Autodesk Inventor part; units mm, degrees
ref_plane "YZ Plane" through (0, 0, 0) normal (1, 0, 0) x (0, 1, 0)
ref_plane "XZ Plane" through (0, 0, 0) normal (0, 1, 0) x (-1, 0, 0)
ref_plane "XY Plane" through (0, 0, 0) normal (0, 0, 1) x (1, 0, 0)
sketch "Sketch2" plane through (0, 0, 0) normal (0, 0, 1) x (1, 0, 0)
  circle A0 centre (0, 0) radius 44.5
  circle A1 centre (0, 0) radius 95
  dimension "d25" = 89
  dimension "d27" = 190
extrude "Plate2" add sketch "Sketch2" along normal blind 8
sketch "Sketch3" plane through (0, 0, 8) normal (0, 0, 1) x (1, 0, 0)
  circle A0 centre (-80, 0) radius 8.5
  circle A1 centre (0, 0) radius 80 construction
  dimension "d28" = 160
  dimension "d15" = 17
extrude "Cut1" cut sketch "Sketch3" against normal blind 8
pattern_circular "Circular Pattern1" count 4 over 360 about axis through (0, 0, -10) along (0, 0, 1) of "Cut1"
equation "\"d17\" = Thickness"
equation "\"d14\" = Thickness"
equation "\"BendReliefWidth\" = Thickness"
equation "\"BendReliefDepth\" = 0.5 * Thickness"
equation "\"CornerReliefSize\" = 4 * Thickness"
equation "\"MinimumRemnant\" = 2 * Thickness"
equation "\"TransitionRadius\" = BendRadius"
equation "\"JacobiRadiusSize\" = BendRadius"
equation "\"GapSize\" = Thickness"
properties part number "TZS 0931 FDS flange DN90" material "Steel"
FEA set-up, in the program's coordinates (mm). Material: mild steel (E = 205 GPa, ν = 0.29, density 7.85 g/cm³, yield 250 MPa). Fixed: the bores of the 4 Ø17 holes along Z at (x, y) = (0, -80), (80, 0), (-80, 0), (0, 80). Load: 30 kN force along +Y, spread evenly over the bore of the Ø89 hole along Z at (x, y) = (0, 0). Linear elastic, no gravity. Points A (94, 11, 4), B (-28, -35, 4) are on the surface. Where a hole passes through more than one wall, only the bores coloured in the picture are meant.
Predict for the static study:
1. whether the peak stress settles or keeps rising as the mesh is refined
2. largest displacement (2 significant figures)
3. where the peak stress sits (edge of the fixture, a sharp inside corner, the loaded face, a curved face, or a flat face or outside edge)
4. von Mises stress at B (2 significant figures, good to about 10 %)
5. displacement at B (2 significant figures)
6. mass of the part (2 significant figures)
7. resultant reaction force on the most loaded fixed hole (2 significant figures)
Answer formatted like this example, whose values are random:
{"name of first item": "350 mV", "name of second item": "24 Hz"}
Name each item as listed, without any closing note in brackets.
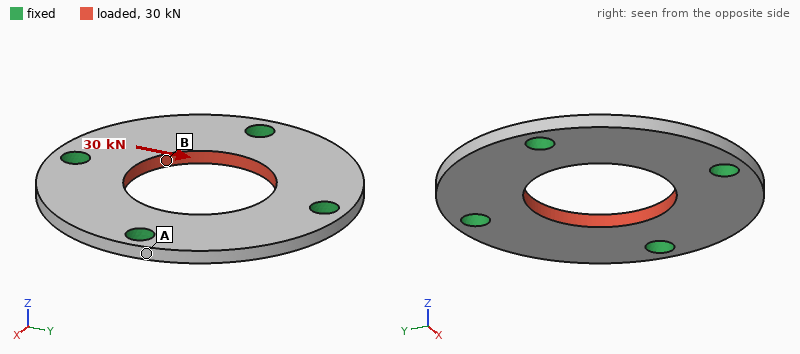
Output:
{"whether the peak stress settles or keeps rising as the mesh is refined": "keeps rising", "largest displacement": "6.6 µm", "where the peak stress sits": "edge of the fixture", "von Mises stress at B": "19 MPa", "displacement at B": "6.0 µm", "mass of the part": "1.3 kg", "resultant reaction force on the most loaded fixed hole": "7.9 kN"}
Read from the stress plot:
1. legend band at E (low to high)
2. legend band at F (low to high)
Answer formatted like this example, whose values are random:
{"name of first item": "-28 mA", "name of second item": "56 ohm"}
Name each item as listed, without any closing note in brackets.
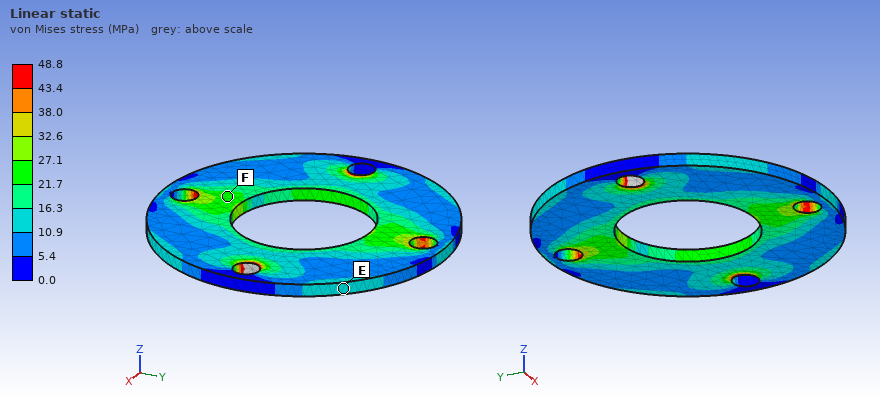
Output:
{"legend band at E": "10.9 to 16.3 MPa", "legend band at F": "21.7 to 27.1 MPa"}
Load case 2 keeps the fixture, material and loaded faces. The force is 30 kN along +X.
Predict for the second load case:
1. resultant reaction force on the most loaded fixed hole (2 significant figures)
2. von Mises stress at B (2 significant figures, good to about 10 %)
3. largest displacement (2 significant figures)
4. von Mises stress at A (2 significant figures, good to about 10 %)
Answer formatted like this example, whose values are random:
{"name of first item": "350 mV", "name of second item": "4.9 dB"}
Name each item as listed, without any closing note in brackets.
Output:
{"resultant reaction force on the most loaded fixed hole": "7.9 kN", "von Mises stress at B": "22 MPa", "largest displacement": "6.6 µm", "von Mises stress at A": "11 MPa"}
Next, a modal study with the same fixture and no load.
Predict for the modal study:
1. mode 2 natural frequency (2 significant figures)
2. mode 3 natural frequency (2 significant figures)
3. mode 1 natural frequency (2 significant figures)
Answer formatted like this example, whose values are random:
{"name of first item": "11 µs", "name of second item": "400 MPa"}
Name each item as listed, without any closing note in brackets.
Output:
{"mode 2 natural frequency": "3100 Hz", "mode 3 natural frequency": "3100 Hz", "mode 1 natural frequency": "3000 Hz"}
